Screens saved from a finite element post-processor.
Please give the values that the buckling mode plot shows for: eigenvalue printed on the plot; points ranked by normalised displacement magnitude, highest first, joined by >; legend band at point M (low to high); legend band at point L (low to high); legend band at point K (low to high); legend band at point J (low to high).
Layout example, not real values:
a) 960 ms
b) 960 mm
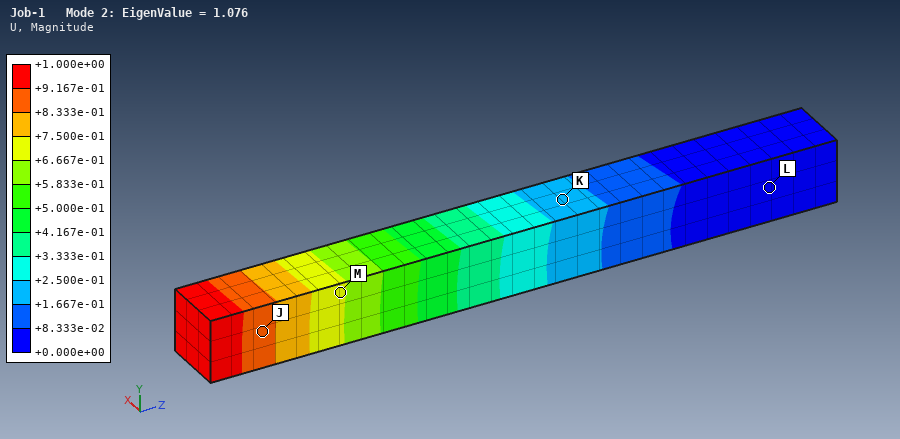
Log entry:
a) 1.076
b) J > M > K > L
c) +6.667e-01 to +7.500e-01
d) +0.000e+00 to +8.333e-02
e) +1.667e-01 to +2.500e-01
f) +8.333e-01 to +9.167e-01
